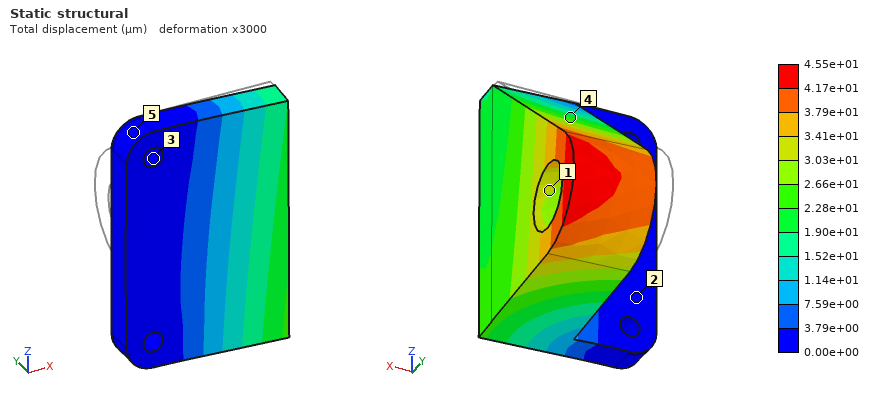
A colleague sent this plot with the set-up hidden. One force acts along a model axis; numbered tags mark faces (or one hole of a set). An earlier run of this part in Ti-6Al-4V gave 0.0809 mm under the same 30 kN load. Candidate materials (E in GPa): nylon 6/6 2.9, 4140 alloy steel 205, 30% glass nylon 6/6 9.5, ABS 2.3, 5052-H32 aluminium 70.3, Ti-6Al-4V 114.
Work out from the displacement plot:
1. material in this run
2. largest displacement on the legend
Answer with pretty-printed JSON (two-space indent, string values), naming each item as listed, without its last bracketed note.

{
  "material in this run": "4140 alloy steel",
  "largest displacement on the legend": "4.55e+01 µm"
}
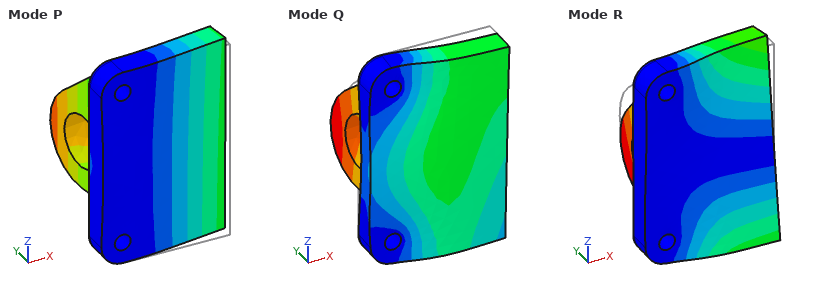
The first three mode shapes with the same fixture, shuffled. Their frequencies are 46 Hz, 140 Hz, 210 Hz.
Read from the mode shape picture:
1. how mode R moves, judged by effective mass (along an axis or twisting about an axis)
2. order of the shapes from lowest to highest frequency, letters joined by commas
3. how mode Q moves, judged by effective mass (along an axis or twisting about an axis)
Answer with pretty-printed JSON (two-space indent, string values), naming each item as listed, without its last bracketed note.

{
  "how mode R moves, judged by effective mass": "along Z",
  "order of the shapes from lowest to highest frequency, letters joined by commas": "P, R, Q",
  "how mode Q moves, judged by effective mass": "along Y"
}
